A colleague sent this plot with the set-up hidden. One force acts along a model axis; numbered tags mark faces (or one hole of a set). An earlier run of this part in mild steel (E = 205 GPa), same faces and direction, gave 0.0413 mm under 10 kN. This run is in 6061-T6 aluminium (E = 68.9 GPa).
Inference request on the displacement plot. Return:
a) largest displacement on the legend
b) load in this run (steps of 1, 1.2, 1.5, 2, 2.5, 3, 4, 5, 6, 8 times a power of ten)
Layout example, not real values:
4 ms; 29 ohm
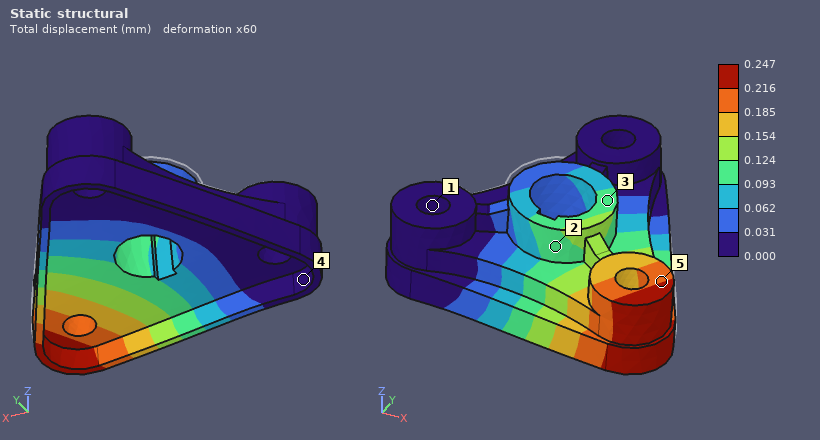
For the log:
0.247 mm; 20 kN
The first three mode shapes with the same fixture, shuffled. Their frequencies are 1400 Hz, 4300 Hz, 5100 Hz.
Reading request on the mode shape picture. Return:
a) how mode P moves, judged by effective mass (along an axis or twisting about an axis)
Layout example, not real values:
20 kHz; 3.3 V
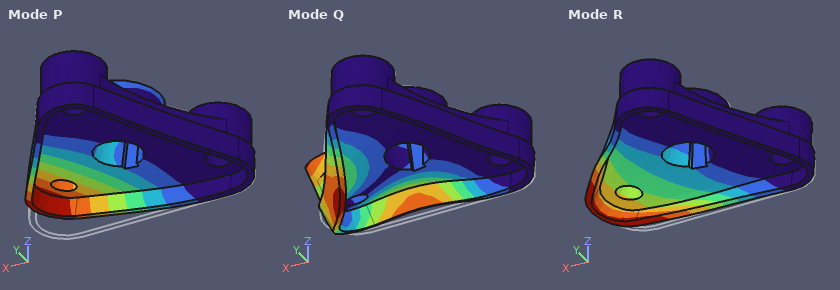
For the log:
along Z
